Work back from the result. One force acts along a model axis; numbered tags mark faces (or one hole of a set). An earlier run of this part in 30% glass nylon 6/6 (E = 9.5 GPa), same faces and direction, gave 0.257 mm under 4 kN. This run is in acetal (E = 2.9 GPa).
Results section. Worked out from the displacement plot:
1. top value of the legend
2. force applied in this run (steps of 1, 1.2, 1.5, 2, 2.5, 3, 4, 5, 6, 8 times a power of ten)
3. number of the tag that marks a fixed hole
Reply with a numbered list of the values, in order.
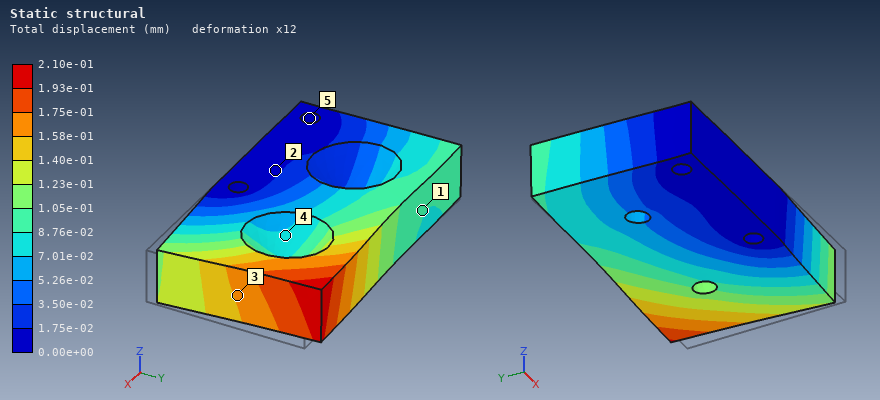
1. 2.10e-01 mm
2. 1 kN
3. 5
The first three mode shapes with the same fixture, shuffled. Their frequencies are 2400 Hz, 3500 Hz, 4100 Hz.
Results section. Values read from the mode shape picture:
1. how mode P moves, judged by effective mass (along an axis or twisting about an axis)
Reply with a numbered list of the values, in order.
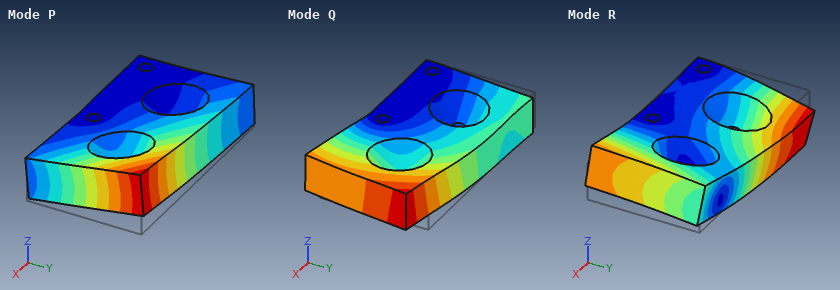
1. along Z
